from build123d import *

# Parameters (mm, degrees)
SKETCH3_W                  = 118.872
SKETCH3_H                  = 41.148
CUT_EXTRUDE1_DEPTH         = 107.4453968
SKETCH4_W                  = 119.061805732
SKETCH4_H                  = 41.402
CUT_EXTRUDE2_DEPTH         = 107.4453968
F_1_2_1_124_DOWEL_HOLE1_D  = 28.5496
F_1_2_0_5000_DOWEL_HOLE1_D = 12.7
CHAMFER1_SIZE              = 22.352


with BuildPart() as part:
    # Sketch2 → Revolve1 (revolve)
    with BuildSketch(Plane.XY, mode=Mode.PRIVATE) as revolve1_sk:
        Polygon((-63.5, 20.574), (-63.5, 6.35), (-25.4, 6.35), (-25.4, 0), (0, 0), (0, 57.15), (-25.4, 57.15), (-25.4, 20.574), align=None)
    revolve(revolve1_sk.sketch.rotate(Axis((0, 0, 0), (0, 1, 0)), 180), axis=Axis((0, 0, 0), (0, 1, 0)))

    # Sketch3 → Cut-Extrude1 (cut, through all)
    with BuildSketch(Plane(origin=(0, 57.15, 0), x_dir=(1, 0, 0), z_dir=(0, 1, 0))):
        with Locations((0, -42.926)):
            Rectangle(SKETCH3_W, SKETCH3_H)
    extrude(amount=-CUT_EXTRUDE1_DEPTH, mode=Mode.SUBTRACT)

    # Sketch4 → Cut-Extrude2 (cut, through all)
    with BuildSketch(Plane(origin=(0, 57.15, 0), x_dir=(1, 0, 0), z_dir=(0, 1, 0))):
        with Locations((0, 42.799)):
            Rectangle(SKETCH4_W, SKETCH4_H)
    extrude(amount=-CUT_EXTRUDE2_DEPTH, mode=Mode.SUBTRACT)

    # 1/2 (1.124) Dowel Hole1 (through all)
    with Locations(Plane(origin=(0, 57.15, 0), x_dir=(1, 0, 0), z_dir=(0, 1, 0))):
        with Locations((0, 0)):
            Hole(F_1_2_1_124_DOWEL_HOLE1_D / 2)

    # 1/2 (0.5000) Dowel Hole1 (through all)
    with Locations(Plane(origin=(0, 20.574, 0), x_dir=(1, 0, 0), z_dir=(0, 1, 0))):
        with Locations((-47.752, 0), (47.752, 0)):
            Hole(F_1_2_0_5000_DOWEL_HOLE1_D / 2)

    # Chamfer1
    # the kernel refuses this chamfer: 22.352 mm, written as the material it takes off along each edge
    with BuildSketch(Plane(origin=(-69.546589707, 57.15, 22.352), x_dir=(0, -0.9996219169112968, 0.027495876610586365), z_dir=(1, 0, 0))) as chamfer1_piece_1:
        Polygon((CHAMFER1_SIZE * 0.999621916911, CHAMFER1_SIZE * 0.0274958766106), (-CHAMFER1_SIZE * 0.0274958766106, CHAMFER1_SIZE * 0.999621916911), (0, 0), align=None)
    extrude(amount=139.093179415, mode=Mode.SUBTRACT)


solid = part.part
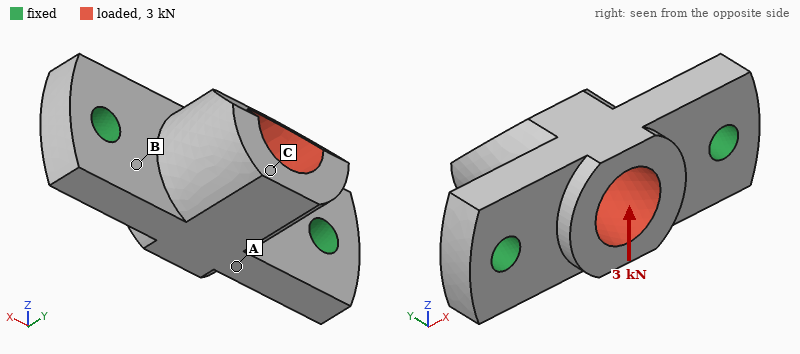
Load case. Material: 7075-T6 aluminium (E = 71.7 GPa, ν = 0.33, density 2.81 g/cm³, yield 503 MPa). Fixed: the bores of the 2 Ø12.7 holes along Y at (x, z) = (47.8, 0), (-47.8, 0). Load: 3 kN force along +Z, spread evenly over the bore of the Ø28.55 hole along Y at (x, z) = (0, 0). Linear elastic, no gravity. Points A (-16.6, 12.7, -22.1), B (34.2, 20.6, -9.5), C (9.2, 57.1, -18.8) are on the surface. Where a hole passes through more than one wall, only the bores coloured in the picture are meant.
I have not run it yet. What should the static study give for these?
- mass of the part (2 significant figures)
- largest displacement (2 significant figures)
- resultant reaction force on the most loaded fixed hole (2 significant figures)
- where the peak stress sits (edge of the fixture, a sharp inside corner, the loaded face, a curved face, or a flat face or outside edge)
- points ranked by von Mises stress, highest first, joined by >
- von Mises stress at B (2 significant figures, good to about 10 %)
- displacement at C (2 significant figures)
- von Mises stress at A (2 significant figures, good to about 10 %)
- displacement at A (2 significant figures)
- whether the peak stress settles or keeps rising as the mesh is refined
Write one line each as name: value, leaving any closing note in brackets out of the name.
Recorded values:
mass of the part: 320 g
largest displacement: 31 µm
resultant reaction force on the most loaded fixed hole: 1.5 kN
where the peak stress sits: edge of the fixture
points ranked by von Mises stress, highest first, joined by >: B > A > C
von Mises stress at B: 14 MPa
displacement at C: 30 µm
von Mises stress at A: 6.9 MPa
displacement at A: 11 µm
whether the peak stress settles or keeps rising as the mesh is refined: keeps rising
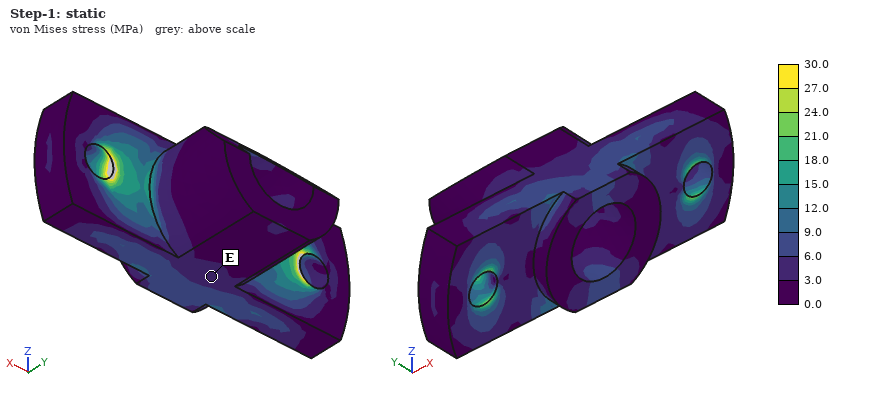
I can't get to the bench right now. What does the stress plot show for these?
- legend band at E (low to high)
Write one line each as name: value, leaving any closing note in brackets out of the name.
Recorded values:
legend band at E: 3.0 to 6.0 MPa
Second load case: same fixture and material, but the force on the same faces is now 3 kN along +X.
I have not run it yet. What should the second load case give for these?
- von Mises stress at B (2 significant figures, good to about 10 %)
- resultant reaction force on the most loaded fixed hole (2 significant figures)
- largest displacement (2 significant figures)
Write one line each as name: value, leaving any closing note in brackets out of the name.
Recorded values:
von Mises stress at B: 3.5 MPa
resultant reaction force on the most loaded fixed hole: 1.6 kN
largest displacement: 7.5 µm
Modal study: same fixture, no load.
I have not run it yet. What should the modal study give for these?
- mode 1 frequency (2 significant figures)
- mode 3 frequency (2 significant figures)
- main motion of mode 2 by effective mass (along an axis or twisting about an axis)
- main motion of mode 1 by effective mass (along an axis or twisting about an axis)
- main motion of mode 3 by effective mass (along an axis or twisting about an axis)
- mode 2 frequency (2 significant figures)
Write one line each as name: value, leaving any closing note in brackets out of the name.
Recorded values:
mode 1 frequency: 4100 Hz
mode 3 frequency: 8700 Hz
main motion of mode 2 by effective mass: along Y
main motion of mode 1 by effective mass: along Z
main motion of mode 3 by effective mass: along X
mode 2 frequency: 6800 Hz
